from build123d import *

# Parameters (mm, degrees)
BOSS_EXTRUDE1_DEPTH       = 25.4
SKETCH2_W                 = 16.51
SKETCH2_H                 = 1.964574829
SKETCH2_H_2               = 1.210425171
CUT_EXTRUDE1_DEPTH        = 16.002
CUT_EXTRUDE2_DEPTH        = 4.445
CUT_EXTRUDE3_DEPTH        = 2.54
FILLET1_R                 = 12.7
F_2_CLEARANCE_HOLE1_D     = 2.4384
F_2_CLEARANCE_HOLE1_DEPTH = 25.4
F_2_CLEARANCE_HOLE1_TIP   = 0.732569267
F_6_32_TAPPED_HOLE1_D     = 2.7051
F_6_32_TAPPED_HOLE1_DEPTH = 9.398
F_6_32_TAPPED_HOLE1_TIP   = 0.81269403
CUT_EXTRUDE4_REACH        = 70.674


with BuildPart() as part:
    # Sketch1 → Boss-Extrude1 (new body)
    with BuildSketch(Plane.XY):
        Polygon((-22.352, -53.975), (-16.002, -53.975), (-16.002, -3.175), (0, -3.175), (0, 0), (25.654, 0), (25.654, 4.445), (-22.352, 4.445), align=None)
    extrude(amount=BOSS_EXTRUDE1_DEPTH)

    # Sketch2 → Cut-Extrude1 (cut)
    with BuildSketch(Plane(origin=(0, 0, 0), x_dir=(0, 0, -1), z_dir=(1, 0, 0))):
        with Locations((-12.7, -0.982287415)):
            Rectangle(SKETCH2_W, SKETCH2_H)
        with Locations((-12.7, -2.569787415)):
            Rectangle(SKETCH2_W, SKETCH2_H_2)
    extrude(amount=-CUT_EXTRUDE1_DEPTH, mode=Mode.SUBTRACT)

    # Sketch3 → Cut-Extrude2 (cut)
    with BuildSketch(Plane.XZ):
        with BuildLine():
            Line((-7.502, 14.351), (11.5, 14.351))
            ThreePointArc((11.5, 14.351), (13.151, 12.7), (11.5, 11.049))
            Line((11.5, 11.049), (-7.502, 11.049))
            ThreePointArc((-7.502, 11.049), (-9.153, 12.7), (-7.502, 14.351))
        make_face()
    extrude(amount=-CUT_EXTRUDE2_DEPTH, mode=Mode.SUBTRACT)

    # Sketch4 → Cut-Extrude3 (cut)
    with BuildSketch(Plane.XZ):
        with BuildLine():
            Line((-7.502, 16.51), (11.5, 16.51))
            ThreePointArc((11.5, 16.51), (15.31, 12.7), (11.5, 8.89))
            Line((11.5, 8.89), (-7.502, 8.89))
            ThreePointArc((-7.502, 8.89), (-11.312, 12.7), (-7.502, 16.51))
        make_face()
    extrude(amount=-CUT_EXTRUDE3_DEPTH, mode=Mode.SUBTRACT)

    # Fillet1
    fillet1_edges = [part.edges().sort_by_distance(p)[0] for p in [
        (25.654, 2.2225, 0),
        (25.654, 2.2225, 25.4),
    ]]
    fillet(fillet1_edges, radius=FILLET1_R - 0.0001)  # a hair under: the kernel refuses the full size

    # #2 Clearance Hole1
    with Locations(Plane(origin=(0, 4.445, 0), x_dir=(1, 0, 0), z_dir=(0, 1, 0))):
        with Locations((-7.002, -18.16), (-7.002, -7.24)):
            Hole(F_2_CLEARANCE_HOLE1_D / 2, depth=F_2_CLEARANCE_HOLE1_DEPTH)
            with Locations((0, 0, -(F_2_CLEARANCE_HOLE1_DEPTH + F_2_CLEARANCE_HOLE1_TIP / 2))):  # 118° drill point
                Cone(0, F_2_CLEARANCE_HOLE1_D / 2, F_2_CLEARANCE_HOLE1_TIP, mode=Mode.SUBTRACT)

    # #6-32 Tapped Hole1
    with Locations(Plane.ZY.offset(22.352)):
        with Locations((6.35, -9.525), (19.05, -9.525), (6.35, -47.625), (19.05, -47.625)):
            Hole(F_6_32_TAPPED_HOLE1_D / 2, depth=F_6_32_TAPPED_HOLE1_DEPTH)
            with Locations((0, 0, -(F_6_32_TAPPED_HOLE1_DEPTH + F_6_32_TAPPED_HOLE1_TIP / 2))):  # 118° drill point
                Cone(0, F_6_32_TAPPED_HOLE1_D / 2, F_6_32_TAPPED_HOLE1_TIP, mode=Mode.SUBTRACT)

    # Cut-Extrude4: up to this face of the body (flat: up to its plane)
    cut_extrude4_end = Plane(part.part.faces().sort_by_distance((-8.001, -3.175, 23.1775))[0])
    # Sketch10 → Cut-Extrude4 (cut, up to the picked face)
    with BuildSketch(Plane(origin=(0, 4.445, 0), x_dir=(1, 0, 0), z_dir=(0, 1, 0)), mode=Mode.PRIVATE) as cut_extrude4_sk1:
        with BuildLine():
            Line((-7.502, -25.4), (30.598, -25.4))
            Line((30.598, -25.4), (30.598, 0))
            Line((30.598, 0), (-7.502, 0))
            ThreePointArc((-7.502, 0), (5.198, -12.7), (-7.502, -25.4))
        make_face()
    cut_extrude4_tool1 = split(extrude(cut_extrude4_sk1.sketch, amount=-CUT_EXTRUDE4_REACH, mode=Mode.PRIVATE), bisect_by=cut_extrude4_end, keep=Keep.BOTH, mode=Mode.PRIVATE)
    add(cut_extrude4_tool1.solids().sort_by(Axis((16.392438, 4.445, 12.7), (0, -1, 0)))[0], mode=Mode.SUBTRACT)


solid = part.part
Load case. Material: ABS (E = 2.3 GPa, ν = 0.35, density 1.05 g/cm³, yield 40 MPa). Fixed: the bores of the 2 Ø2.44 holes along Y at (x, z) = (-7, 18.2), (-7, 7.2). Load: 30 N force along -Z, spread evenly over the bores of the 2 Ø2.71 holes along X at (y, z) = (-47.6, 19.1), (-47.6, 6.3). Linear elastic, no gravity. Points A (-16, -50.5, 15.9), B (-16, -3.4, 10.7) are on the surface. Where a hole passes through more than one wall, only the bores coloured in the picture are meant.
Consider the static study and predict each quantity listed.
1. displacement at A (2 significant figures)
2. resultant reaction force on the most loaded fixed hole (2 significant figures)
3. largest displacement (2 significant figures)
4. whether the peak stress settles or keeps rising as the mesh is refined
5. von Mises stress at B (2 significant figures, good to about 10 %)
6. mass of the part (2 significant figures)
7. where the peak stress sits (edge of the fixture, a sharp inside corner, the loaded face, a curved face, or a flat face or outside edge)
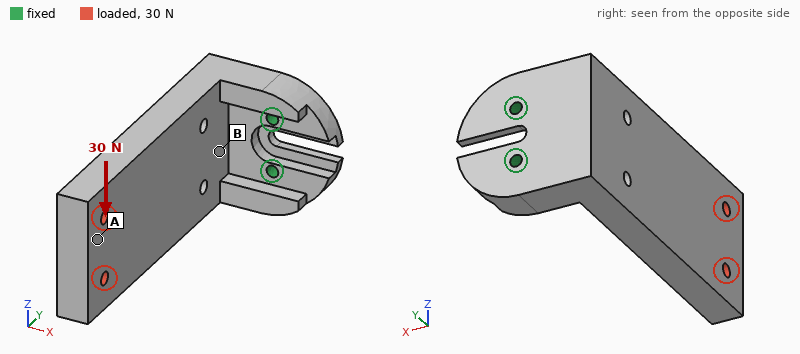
0.62 mm
83 N
0.68 mm
keeps rising
3.2 MPa
12 g
edge of the fixture
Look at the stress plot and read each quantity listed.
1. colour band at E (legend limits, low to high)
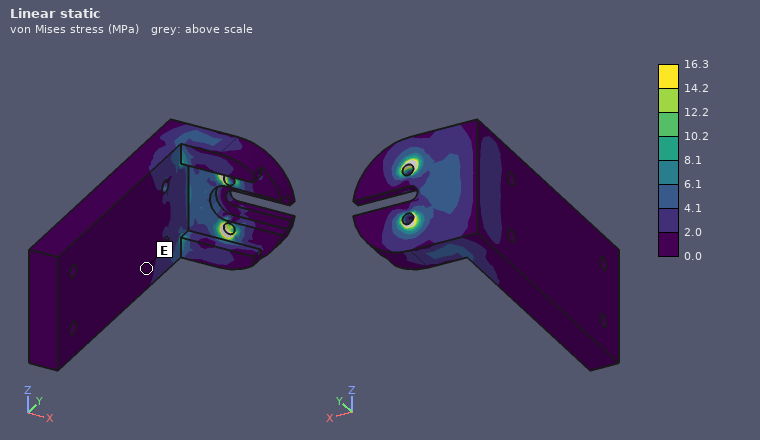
0.0 to 2.0 MPa
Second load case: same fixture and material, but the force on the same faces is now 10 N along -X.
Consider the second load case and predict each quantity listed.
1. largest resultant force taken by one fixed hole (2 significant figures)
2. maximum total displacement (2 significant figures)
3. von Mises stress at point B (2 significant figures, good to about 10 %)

7.8 N
0.83 mm
2.1 MPa
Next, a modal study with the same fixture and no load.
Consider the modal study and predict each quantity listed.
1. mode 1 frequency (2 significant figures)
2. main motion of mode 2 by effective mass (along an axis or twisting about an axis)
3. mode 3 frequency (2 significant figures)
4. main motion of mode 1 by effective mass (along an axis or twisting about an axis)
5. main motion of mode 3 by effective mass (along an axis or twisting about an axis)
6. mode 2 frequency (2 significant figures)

310 Hz
along Z
1600 Hz
along X
along Y
570 Hz
